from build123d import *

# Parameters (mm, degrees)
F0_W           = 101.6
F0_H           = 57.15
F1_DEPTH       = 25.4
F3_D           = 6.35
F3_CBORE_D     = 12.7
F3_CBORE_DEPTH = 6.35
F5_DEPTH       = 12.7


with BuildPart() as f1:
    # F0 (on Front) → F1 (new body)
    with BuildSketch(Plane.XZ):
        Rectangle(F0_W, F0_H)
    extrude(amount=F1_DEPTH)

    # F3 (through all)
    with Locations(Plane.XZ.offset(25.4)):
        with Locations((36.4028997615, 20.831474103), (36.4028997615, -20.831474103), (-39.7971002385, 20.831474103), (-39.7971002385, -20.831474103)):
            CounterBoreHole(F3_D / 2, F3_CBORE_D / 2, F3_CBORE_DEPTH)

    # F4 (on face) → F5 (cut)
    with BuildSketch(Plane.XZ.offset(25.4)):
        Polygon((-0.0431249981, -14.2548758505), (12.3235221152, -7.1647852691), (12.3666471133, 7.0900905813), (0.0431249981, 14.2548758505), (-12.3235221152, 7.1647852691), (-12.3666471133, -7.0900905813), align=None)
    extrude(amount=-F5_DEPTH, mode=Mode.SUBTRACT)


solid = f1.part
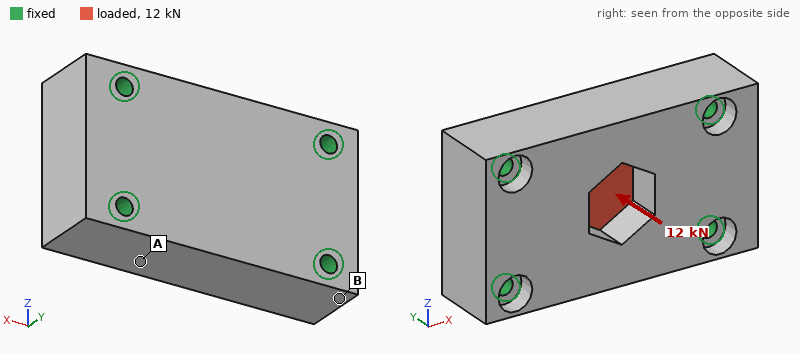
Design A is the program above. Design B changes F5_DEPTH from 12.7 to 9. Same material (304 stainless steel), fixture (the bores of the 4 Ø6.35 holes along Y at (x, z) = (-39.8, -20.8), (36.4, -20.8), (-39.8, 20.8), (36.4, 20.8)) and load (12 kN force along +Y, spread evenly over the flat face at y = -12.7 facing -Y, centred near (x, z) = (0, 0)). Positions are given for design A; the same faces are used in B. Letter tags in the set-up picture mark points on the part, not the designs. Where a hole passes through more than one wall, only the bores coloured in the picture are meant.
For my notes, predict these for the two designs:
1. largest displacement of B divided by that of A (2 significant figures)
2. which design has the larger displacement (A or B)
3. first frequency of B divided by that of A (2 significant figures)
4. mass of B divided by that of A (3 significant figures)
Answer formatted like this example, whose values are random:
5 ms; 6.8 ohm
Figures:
0.91; A; 0.99; 1.01
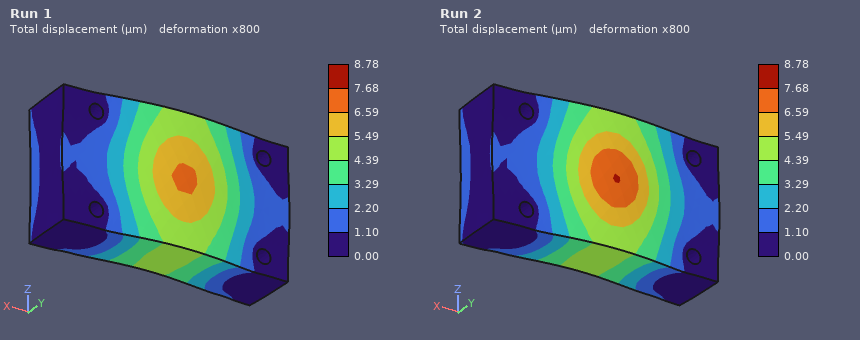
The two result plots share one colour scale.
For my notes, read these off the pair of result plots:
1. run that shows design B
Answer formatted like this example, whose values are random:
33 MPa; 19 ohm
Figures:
Run 1
